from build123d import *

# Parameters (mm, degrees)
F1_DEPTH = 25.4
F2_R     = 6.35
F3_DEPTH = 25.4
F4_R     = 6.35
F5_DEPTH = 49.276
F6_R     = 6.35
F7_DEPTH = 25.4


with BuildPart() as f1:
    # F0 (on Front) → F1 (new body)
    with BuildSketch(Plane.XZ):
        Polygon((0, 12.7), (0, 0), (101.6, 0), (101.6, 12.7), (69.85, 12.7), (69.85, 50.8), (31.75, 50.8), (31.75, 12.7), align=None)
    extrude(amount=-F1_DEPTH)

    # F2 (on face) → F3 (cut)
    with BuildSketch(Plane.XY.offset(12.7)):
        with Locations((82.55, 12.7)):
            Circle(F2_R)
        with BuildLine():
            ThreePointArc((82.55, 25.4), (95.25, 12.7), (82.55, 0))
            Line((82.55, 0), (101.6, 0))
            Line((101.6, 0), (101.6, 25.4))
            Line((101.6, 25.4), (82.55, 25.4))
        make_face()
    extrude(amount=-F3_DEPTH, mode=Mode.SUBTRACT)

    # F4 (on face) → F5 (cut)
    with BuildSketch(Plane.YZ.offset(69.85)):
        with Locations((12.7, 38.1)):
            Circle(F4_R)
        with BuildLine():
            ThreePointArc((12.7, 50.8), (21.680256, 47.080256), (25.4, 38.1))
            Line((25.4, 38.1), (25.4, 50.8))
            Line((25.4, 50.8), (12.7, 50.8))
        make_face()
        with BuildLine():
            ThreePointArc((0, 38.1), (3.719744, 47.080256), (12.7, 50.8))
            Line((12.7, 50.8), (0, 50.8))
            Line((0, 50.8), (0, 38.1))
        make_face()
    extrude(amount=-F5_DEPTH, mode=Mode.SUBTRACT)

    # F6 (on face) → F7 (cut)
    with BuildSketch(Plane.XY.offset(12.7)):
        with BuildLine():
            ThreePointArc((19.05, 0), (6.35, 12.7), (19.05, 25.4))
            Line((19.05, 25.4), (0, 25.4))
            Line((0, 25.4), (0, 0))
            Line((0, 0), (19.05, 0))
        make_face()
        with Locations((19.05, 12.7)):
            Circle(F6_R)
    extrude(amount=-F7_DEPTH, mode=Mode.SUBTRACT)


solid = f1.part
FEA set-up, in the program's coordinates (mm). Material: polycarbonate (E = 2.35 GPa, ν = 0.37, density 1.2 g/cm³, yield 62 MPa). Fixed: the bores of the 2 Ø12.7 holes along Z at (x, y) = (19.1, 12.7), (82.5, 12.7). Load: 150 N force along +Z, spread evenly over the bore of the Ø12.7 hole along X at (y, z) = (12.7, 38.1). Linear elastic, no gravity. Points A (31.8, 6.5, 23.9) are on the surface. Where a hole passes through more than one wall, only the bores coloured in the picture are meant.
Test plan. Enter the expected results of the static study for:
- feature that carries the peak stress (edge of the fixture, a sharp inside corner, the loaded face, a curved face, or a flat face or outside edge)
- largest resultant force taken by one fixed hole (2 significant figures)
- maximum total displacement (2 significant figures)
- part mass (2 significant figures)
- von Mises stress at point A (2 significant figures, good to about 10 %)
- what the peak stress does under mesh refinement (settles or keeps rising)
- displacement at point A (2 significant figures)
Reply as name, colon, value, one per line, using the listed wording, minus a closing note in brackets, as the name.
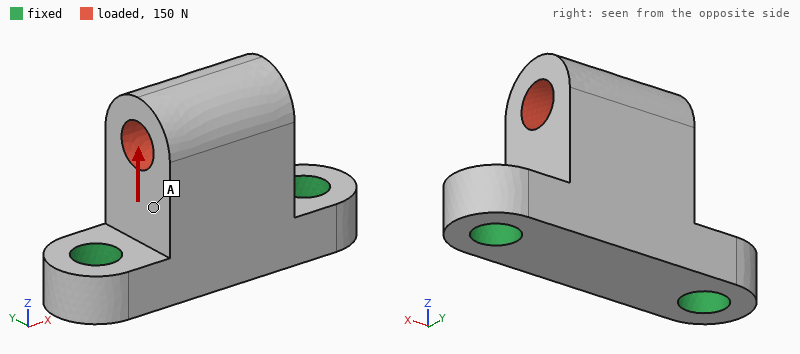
feature that carries the peak stress: edge of the fixture
largest resultant force taken by one fixed hole: 80 N
maximum total displacement: 9.5 µm
part mass: 64 g
von Mises stress at point A: 0.22 MPa
what the peak stress does under mesh refinement: keeps rising
displacement at point A: 6.5 µm
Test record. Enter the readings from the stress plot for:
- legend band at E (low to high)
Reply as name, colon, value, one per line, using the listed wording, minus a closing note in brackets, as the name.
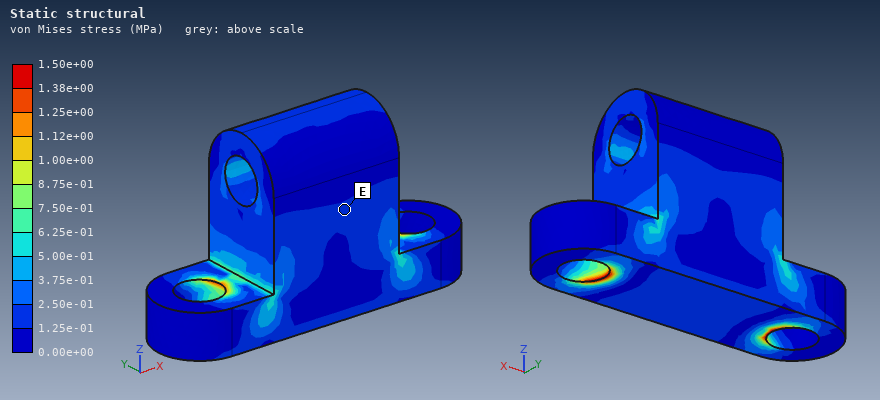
legend band at E: 1.25e-01 to 2.50e-01 MPa
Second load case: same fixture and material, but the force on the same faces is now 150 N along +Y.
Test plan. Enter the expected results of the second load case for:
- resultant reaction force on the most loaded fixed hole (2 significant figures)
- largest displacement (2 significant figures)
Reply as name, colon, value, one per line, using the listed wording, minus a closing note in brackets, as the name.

resultant reaction force on the most loaded fixed hole: 75 N
largest displacement: 0.14 mm
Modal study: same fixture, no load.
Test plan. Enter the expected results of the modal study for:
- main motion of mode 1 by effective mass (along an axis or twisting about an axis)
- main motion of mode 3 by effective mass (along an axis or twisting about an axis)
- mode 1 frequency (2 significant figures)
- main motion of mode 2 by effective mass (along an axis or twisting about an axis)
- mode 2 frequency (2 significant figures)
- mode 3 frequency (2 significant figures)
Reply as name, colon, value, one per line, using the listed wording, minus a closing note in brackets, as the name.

main motion of mode 1 by effective mass: along Y
main motion of mode 3 by effective mass: along Z
mode 1 frequency: 1300 Hz
main motion of mode 2 by effective mass: along X
mode 2 frequency: 2900 Hz
mode 3 frequency: 3400 Hz
